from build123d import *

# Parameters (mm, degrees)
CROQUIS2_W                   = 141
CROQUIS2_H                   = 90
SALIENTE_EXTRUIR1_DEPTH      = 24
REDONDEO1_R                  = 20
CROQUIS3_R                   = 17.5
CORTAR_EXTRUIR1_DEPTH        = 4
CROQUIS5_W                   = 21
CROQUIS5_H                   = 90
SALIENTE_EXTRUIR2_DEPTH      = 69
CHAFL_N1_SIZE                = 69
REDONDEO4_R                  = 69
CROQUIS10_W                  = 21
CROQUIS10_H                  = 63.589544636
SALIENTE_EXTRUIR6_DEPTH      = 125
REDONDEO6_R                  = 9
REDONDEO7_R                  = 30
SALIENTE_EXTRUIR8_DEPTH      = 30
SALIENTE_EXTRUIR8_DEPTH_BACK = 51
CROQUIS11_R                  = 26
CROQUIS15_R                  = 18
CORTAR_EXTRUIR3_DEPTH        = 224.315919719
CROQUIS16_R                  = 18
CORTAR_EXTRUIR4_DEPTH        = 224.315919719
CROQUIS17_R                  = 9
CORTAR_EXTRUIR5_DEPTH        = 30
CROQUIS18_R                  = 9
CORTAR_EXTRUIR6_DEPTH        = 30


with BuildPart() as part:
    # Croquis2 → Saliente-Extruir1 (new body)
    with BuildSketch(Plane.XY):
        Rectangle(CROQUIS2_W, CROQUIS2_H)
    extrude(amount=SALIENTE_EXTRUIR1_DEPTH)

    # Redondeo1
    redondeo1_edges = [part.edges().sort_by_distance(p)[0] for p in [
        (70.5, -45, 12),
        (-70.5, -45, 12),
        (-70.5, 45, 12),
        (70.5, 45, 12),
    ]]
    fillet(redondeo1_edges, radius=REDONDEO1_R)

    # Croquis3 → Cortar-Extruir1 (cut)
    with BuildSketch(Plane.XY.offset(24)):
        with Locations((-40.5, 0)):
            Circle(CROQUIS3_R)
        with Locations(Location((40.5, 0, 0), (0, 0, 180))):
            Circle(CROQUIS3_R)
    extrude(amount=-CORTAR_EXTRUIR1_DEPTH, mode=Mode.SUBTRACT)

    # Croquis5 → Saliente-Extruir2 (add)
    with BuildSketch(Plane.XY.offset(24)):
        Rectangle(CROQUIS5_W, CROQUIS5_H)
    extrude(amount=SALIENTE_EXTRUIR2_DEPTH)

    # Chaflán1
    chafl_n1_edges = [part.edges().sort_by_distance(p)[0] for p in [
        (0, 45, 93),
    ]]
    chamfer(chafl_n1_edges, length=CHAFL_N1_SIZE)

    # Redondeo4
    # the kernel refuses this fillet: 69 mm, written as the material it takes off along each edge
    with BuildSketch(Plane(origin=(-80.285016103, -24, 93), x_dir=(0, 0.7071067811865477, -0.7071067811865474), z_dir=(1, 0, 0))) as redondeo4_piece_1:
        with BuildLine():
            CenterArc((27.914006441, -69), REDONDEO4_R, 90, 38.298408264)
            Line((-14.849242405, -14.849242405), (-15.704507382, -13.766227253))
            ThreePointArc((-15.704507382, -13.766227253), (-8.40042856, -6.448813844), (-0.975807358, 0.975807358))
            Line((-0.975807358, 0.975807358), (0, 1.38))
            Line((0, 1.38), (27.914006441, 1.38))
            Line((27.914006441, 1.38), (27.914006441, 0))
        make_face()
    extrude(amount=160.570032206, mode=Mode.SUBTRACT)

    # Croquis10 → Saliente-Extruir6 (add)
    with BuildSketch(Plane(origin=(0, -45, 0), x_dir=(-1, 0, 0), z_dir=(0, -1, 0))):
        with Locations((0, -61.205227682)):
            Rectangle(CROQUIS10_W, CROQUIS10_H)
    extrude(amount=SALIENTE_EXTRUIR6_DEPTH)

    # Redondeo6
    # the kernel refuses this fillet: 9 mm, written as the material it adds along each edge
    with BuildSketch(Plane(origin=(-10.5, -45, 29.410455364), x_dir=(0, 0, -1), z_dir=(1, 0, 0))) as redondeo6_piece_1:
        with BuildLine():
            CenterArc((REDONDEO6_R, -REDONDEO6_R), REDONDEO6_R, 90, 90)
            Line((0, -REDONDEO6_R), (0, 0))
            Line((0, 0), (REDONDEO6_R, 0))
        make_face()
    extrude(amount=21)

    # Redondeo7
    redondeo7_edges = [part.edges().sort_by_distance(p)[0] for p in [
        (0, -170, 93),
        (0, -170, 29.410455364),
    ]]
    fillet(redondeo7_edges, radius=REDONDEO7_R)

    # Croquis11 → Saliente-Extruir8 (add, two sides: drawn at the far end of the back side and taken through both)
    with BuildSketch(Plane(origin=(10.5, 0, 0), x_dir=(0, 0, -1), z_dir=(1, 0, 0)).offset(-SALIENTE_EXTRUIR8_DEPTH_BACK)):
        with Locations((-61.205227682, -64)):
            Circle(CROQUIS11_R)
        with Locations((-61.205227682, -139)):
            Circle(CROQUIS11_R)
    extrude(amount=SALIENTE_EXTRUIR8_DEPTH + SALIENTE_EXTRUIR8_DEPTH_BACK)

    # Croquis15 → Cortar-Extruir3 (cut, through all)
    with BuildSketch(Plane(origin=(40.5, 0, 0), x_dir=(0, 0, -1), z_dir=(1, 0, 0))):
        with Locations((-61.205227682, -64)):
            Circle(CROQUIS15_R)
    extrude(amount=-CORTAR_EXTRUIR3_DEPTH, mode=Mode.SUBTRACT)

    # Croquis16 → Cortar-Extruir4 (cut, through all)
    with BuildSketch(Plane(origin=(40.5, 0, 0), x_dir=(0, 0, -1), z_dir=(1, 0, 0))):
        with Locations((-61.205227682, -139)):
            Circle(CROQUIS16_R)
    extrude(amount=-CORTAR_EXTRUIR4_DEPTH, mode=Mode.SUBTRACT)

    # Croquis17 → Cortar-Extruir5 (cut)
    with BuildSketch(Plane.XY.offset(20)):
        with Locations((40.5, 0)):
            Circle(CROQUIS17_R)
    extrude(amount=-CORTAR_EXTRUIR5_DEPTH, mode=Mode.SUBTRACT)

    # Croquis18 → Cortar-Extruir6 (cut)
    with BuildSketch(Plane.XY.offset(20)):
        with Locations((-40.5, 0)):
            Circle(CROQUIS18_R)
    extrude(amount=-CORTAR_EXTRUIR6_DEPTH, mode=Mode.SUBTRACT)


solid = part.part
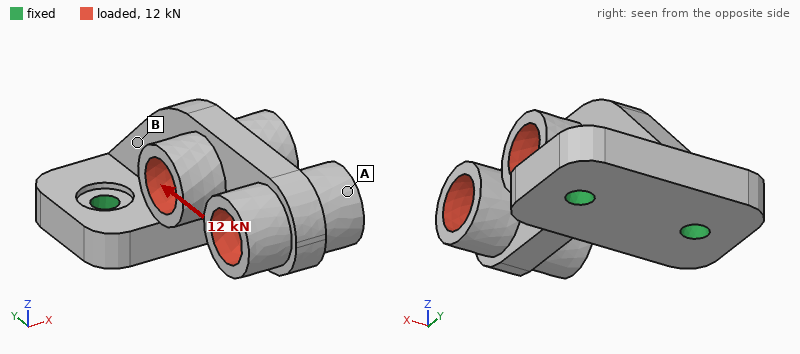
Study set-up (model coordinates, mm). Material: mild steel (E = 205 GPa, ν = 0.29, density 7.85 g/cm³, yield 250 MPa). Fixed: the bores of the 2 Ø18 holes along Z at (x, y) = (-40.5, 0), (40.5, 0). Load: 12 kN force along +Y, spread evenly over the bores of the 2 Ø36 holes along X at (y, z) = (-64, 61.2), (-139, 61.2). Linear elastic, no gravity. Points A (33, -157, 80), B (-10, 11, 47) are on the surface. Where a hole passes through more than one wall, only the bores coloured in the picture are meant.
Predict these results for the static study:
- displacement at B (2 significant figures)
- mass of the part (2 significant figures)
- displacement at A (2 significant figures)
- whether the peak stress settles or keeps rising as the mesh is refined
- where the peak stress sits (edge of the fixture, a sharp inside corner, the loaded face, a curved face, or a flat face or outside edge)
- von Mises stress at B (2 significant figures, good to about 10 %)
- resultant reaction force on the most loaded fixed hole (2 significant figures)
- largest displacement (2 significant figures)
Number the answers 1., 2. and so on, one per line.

1. 19 µm
2. 4.8 kg
3. 95 µm
4. keeps rising
5. edge of the fixture
6. 19 MPa
7. 6.0 kN
8. 99 µm
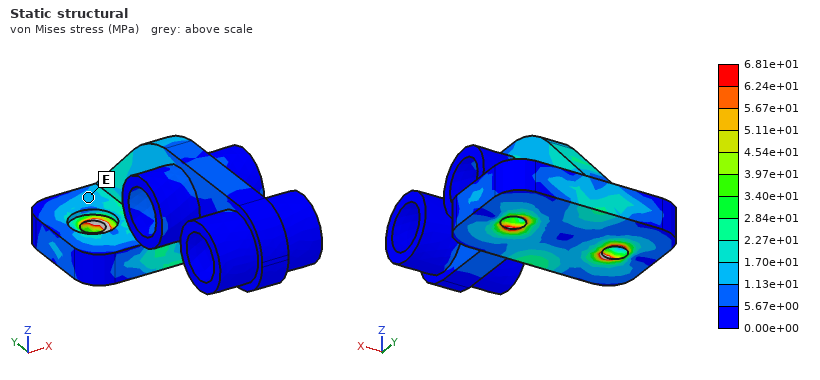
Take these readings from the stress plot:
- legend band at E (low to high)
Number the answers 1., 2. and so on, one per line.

1. 1.13e+01 to 1.70e+01 MPa
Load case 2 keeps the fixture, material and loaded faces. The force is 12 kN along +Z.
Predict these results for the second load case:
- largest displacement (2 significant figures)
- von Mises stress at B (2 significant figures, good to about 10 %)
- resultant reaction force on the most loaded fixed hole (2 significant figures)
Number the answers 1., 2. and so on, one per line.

1. 0.27 mm
2. 38 MPa
3. 7.1 kN
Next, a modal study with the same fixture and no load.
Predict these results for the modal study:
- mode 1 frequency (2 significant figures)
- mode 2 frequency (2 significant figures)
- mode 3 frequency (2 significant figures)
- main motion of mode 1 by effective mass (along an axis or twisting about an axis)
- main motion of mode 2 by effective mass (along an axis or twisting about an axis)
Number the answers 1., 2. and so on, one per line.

1. 570 Hz
2. 860 Hz
3. 1500 Hz
4. along X
5. along Z
